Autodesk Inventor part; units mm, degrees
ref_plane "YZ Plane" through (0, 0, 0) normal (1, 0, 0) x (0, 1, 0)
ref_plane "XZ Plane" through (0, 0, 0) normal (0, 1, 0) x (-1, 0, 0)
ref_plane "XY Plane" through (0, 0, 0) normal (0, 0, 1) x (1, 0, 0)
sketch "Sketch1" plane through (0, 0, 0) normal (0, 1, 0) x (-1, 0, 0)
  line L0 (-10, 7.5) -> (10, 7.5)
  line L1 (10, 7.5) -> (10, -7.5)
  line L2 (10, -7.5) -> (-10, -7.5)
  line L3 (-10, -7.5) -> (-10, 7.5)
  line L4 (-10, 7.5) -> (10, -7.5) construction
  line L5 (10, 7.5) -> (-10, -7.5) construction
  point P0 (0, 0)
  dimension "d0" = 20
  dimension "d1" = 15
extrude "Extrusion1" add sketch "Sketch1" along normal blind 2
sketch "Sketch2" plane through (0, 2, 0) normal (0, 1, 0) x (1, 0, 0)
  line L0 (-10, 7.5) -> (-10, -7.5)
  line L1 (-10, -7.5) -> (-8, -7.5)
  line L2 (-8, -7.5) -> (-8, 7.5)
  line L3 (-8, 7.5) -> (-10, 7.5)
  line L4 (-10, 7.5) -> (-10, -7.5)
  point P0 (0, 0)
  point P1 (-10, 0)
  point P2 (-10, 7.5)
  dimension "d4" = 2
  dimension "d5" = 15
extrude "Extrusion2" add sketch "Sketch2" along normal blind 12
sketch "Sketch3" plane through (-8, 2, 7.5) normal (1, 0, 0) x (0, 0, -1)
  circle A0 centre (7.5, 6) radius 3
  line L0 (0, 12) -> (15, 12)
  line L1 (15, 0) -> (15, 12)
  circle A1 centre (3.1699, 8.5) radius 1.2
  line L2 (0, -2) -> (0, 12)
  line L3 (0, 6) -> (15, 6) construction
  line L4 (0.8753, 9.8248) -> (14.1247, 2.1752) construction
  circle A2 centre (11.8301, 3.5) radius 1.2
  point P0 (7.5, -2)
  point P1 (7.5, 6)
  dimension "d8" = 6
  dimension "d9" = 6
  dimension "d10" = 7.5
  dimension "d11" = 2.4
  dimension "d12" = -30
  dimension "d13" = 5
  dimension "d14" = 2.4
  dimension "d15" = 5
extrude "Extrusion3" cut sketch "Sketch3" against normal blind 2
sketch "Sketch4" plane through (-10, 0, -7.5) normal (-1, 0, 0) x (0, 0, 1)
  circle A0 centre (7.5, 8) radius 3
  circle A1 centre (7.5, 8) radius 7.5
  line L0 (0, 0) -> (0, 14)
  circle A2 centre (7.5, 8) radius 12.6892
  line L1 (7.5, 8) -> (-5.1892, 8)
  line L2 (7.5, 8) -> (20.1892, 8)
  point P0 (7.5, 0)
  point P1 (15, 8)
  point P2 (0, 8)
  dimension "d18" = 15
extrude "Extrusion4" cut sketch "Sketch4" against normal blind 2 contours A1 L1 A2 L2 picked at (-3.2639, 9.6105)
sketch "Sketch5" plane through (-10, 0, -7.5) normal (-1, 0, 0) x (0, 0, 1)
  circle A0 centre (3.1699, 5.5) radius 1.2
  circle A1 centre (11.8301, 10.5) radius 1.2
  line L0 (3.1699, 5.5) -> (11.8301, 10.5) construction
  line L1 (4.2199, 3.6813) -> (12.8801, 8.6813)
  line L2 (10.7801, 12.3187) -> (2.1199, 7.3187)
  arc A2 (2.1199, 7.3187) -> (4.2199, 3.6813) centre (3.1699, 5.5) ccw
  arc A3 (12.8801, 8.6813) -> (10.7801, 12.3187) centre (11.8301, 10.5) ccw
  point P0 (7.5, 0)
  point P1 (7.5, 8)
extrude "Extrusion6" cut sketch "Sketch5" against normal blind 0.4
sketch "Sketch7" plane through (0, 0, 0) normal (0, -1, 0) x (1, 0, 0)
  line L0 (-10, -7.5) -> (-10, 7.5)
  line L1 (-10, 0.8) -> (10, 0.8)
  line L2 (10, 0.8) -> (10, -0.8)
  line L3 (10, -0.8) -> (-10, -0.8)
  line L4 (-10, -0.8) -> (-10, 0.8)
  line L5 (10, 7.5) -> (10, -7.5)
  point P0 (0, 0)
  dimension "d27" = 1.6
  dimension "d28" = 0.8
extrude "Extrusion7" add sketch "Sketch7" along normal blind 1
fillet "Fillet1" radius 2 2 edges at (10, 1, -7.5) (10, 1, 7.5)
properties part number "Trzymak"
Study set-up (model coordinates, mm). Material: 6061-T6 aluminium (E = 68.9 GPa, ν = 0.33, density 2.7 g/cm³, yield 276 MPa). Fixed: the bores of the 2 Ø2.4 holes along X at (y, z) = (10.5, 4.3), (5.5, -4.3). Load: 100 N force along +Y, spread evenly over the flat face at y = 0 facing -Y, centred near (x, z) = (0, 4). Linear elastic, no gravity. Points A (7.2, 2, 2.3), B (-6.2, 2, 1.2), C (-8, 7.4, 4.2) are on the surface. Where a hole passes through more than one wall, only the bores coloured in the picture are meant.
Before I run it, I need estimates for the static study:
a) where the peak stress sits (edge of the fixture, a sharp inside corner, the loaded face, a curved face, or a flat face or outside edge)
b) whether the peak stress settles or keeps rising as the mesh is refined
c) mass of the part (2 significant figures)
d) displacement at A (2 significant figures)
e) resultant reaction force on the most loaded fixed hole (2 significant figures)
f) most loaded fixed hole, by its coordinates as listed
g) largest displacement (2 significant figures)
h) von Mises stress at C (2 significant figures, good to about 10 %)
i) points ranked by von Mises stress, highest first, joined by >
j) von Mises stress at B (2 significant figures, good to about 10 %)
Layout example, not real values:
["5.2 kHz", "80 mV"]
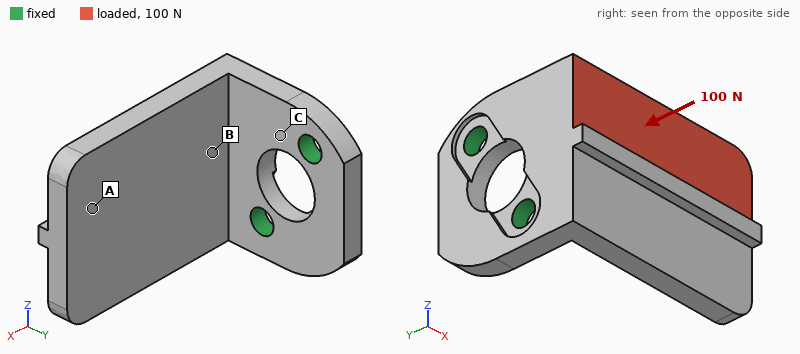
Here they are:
["edge of the fixture", "keeps rising", "2.4 g", "0.22 mm", "83 N", "(10.5, 4.3)", "0.28 mm", "99 MPa", "C > B > A", "57 MPa"]
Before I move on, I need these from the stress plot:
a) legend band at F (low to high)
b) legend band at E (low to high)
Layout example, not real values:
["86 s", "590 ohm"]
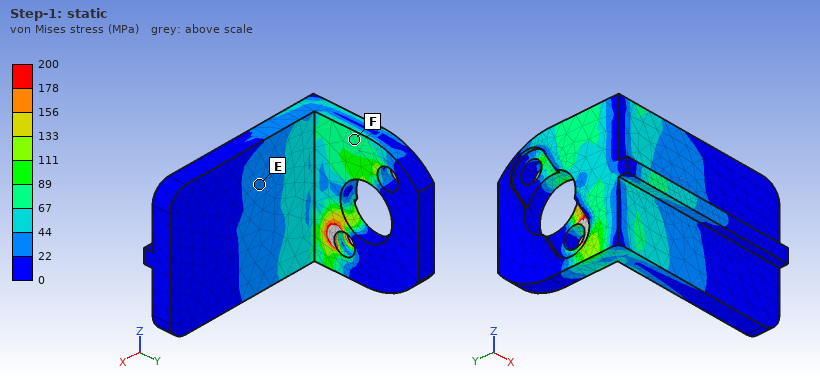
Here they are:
["67 to 89 MPa", "22 to 44 MPa"]
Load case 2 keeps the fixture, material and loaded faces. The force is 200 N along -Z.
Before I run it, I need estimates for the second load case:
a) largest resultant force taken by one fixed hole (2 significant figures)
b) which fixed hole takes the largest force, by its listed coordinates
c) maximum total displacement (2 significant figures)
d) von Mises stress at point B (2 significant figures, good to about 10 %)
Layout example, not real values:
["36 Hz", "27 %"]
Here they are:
["230 N", "(5.5, -4.3)", "0.18 mm", "35 MPa"]
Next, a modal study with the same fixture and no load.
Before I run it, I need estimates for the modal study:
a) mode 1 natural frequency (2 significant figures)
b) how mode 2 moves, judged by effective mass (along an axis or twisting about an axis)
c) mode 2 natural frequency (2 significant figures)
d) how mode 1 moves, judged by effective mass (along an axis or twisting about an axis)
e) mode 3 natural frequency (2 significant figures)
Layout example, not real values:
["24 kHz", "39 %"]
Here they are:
["2900 Hz", "along Z", "5500 Hz", "along Y", "12 kHz"]
